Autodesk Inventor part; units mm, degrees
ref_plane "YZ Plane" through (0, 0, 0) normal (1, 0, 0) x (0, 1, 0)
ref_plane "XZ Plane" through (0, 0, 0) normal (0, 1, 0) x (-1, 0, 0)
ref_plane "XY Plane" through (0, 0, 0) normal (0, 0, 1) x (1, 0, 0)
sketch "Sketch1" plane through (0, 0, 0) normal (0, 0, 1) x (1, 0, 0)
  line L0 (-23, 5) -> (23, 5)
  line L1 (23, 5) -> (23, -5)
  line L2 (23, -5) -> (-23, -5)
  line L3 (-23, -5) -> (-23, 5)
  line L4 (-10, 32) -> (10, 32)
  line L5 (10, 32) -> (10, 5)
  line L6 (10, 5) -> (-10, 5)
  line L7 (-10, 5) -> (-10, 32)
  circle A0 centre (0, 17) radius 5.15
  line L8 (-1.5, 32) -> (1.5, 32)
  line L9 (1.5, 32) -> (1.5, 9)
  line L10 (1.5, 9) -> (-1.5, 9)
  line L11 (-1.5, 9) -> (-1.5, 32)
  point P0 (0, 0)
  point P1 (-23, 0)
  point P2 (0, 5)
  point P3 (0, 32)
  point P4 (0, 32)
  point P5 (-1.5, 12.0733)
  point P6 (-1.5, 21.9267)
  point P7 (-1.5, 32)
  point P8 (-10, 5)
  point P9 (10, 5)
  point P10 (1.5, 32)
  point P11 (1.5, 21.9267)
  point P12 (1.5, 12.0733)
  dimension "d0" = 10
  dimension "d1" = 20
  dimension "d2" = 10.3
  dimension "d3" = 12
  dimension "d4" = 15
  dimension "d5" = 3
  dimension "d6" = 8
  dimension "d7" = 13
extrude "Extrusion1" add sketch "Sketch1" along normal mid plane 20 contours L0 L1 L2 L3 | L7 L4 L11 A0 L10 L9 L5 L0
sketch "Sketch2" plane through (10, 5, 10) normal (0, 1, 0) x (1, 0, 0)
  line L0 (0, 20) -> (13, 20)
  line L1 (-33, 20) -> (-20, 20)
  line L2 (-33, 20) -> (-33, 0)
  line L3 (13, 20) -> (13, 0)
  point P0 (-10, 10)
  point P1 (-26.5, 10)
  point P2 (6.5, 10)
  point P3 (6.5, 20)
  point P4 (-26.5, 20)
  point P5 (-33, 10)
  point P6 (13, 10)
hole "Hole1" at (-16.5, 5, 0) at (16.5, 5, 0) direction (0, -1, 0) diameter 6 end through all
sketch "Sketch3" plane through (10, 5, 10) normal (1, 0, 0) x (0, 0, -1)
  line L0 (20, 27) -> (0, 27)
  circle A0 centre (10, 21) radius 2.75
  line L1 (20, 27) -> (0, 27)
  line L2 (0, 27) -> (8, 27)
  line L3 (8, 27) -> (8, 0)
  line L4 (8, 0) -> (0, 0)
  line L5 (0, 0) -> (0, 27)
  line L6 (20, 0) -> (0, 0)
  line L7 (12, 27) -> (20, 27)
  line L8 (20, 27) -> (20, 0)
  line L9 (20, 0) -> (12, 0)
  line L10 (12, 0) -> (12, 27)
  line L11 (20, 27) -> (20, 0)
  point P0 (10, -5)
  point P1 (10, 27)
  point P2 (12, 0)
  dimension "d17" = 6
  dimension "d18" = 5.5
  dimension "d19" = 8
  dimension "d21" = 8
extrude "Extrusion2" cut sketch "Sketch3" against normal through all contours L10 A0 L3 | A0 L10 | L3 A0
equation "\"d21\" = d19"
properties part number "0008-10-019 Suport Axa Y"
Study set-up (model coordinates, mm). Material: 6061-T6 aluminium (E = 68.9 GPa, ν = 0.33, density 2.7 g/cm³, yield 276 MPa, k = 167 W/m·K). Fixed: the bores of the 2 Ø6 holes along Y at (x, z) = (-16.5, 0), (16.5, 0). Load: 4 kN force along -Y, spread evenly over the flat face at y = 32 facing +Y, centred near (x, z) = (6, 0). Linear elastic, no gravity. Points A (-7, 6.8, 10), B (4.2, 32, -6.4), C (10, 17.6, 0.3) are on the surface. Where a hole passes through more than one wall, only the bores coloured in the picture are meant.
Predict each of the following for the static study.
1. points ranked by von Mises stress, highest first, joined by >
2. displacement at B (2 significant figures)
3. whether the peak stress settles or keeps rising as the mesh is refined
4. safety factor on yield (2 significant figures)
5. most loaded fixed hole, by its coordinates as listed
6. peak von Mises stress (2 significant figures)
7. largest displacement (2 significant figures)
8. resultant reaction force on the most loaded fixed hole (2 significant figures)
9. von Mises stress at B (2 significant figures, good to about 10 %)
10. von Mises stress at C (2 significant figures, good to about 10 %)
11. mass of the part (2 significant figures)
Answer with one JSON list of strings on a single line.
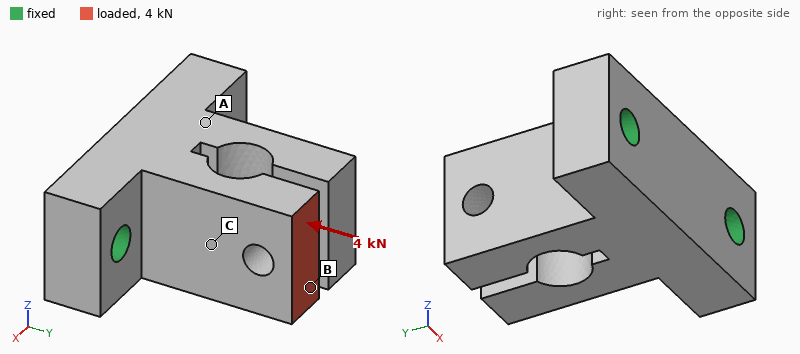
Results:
["C > B > A", "62 µm", "settles", "1.8", "(16.5, 0)", "150 MPa", "71 µm", "2.9 kN", "29 MPa", "41 MPa", "45 g"]
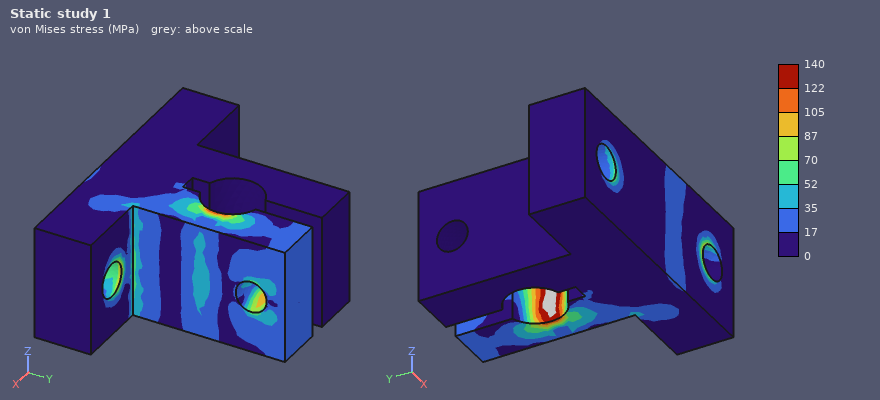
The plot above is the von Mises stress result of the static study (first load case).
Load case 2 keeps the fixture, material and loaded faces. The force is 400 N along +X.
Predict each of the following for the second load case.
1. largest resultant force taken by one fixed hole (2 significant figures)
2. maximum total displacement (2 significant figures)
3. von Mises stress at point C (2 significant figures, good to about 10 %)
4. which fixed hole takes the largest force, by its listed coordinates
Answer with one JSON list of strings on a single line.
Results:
["570 N", "90 µm", "60 MPa", "(-16.5, 0)"]
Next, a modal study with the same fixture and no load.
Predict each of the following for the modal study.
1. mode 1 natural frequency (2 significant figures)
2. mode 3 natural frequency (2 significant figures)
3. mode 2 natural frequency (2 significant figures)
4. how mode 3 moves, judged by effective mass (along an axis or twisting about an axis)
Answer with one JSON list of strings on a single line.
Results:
["6900 Hz", "7600 Hz", "6900 Hz", "along Z"]
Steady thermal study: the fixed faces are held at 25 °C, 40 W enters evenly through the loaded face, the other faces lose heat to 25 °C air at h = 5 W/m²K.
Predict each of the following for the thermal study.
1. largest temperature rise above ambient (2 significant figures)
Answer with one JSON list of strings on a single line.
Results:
["59 K"]
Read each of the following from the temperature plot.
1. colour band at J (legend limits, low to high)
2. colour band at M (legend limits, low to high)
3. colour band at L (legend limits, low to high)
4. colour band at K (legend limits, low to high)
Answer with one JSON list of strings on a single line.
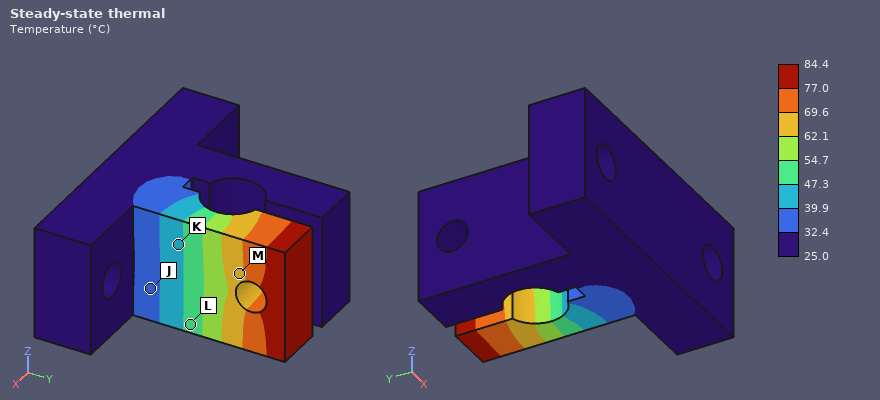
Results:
["32.4 to 39.9 °C", "62.1 to 69.6 °C", "47.3 to 54.7 °C", "39.9 to 47.3 °C"]
